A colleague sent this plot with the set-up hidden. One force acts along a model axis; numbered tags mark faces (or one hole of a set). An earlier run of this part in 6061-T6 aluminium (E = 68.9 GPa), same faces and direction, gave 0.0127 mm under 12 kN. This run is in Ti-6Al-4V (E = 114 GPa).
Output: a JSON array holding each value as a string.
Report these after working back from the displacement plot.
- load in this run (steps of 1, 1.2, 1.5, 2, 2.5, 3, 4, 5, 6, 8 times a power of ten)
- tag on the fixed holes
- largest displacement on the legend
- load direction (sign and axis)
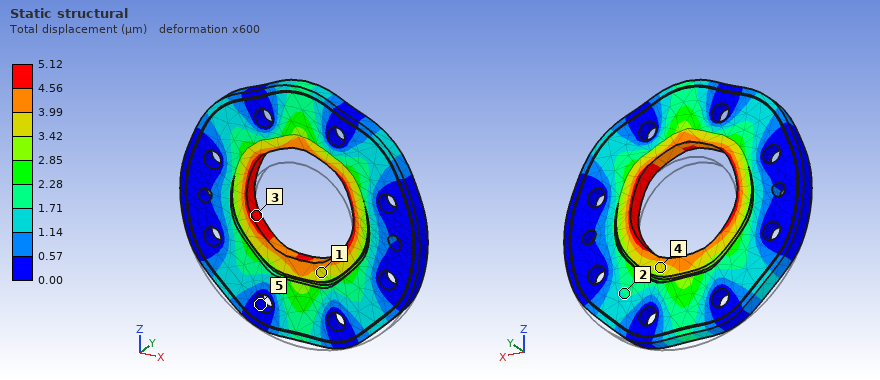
["8 kN", "5", "5.12 µm", "+Z"]
